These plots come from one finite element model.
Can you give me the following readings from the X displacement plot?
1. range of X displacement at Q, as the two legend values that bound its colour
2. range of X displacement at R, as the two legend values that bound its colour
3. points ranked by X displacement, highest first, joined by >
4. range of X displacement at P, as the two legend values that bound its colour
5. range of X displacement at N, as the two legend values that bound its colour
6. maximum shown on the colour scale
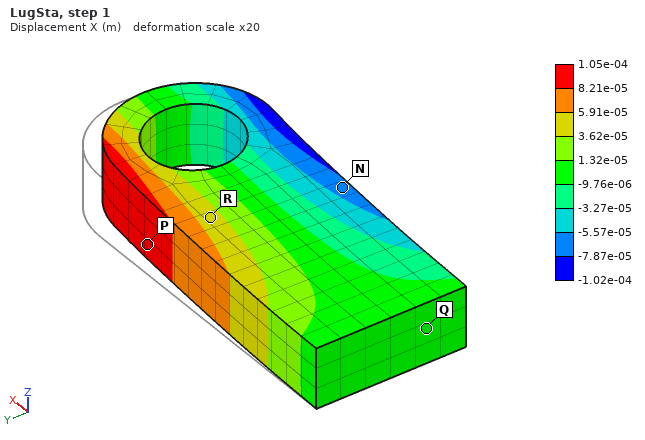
-9.76e-06 to 1.32e-05 m
3.62e-05 to 5.91e-05 m
P > R > Q > N
8.21e-05 to 1.05e-04 m
-7.87e-05 to -5.57e-05 m
1.05e-04 m
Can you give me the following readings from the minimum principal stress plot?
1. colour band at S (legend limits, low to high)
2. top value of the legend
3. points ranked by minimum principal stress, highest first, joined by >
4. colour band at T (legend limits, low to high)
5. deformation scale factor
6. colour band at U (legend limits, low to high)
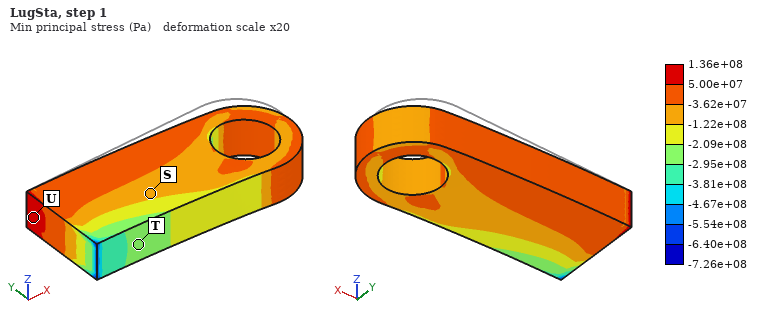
-1.22e+08 to -3.62e+07 Pa
1.36e+08 Pa
U > S > T
-2.95e+08 to -2.09e+08 Pa
20
5.00e+07 to 1.36e+08 Pa
